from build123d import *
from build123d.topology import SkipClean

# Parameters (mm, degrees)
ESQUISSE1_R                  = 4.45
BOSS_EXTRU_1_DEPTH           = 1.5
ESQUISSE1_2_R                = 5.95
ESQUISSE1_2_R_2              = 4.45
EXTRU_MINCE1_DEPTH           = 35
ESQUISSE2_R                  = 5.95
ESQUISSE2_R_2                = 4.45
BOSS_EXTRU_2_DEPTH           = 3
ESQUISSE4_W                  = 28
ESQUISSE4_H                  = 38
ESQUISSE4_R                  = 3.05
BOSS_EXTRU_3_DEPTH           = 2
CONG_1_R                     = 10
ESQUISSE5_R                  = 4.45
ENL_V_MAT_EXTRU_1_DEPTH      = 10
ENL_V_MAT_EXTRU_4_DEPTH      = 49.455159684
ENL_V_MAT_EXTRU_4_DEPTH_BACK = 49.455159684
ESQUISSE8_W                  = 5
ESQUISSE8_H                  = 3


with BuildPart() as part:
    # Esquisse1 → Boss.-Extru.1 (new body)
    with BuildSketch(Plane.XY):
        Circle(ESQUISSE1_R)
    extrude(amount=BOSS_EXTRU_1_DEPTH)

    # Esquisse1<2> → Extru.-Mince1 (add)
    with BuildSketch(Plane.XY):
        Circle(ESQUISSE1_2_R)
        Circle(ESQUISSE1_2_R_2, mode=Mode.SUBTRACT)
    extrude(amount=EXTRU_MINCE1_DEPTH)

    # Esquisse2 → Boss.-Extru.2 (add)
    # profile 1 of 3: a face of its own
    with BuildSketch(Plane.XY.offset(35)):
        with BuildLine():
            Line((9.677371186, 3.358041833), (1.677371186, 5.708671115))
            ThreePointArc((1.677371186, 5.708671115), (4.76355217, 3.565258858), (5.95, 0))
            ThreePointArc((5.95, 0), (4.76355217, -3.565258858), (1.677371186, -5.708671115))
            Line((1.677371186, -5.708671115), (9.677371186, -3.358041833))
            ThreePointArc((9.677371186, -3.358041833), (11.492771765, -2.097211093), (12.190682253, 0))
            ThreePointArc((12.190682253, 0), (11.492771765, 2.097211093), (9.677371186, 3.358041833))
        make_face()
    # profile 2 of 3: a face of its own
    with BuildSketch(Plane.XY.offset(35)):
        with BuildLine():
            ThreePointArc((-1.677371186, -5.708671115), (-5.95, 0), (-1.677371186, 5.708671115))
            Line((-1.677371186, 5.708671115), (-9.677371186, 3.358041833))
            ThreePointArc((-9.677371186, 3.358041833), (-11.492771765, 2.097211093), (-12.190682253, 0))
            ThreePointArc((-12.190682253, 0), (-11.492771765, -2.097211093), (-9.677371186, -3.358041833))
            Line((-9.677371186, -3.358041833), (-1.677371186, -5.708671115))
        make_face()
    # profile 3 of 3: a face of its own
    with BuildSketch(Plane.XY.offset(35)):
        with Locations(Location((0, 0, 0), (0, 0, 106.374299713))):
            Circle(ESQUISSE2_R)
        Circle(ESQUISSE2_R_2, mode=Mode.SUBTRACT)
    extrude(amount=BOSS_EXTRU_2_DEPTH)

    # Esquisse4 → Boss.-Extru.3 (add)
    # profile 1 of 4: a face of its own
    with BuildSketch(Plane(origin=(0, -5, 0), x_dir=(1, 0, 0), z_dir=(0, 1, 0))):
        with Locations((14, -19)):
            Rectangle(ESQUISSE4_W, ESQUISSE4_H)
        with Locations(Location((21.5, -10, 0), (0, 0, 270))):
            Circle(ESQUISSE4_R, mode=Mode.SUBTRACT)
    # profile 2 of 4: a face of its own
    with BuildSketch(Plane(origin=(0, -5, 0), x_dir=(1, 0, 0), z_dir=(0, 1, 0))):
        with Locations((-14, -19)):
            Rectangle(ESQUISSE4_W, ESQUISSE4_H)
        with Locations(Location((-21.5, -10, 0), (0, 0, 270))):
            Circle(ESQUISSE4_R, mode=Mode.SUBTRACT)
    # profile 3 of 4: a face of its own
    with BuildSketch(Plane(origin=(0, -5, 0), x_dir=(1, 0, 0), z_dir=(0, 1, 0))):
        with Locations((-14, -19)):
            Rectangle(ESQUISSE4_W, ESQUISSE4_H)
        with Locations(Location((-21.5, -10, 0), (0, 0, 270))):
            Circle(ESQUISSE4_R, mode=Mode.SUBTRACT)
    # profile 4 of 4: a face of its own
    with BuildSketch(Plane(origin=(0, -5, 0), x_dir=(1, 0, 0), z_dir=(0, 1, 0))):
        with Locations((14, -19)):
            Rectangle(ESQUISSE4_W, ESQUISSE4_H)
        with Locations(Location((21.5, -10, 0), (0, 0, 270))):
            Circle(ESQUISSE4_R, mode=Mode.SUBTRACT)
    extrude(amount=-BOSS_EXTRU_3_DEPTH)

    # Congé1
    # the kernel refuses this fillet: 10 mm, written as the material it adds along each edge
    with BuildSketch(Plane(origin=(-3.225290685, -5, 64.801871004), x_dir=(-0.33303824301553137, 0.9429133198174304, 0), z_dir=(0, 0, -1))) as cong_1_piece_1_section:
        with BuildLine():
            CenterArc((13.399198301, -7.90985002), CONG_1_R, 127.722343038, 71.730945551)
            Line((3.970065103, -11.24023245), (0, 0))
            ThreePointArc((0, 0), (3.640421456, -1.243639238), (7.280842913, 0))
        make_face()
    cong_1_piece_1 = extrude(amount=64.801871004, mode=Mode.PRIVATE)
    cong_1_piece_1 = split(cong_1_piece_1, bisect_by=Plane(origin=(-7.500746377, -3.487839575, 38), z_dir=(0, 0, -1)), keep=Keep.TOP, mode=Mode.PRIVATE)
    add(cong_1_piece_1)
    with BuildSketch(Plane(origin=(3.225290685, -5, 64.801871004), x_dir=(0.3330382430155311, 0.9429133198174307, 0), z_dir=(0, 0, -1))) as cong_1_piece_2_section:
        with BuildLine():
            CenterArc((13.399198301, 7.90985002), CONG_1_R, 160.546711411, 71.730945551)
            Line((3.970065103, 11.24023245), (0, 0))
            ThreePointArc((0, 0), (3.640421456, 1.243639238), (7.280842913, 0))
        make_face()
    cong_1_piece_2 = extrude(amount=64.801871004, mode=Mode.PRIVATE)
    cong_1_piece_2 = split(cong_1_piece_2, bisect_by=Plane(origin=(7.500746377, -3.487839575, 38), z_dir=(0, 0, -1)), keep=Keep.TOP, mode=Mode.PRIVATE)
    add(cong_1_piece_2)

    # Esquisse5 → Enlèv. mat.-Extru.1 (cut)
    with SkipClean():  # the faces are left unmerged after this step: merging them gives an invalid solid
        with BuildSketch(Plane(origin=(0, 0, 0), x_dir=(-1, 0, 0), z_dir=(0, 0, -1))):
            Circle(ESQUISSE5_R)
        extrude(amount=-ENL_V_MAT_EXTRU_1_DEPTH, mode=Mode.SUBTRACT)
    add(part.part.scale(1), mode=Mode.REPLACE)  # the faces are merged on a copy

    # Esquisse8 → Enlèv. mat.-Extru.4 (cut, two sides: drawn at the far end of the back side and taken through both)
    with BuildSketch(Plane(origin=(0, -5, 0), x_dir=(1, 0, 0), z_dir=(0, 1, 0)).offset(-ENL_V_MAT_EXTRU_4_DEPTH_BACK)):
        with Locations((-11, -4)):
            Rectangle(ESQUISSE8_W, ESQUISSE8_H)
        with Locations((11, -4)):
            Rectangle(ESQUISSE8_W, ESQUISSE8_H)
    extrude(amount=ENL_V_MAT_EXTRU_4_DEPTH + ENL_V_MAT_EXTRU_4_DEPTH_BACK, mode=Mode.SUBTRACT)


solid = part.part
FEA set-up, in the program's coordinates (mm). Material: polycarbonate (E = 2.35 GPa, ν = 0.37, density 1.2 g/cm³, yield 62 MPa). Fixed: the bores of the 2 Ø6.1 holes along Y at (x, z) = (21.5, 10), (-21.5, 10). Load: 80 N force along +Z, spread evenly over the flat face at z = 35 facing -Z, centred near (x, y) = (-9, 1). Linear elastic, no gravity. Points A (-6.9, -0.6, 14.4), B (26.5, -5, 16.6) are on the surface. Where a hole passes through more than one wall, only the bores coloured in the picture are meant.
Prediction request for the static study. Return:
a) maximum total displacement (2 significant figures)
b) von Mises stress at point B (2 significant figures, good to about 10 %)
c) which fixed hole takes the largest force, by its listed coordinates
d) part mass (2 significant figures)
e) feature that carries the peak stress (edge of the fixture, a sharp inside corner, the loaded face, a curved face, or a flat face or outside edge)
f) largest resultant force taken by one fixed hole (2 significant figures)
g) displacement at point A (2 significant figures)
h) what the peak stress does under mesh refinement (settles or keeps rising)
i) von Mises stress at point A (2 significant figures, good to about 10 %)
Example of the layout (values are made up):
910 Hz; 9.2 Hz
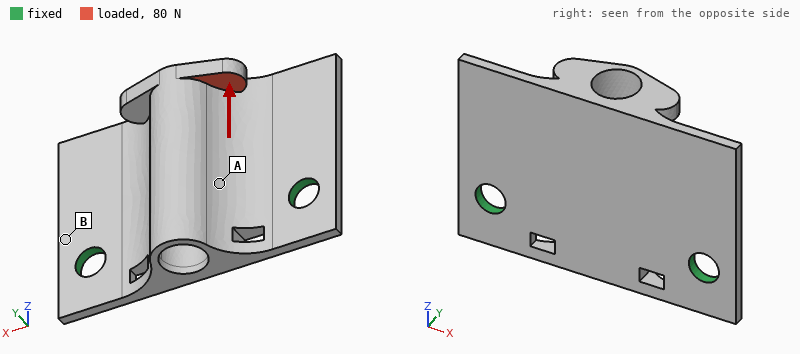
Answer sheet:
0.81 mm; 7.6 MPa; (-21.5, 10); 9.0 g; a sharp inside corner; 58 N; 0.17 mm; keeps rising; 2.4 MPa
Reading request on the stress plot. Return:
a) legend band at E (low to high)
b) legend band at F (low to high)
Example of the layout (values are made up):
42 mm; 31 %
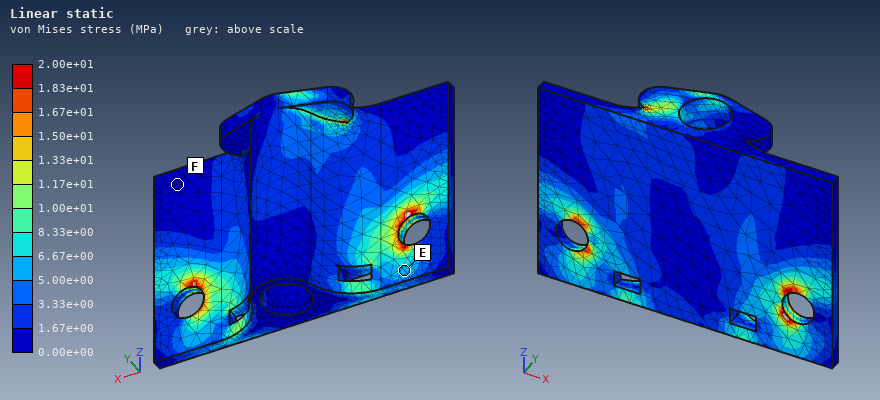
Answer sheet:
5.00e+00 to 6.67e+00 MPa; 0.00e+00 to 1.67e+00 MPa
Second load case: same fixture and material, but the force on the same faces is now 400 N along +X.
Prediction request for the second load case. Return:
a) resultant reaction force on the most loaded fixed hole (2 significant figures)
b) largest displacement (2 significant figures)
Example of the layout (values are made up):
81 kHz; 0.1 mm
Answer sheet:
320 N; 0.67 mm
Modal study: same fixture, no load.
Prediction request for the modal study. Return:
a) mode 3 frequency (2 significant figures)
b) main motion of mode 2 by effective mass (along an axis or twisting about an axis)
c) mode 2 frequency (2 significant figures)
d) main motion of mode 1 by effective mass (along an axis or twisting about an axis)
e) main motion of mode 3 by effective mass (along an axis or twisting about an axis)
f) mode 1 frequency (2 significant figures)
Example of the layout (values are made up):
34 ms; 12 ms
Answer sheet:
2000 Hz; twisting about Z; 1700 Hz; along Y; along Y; 540 Hz
